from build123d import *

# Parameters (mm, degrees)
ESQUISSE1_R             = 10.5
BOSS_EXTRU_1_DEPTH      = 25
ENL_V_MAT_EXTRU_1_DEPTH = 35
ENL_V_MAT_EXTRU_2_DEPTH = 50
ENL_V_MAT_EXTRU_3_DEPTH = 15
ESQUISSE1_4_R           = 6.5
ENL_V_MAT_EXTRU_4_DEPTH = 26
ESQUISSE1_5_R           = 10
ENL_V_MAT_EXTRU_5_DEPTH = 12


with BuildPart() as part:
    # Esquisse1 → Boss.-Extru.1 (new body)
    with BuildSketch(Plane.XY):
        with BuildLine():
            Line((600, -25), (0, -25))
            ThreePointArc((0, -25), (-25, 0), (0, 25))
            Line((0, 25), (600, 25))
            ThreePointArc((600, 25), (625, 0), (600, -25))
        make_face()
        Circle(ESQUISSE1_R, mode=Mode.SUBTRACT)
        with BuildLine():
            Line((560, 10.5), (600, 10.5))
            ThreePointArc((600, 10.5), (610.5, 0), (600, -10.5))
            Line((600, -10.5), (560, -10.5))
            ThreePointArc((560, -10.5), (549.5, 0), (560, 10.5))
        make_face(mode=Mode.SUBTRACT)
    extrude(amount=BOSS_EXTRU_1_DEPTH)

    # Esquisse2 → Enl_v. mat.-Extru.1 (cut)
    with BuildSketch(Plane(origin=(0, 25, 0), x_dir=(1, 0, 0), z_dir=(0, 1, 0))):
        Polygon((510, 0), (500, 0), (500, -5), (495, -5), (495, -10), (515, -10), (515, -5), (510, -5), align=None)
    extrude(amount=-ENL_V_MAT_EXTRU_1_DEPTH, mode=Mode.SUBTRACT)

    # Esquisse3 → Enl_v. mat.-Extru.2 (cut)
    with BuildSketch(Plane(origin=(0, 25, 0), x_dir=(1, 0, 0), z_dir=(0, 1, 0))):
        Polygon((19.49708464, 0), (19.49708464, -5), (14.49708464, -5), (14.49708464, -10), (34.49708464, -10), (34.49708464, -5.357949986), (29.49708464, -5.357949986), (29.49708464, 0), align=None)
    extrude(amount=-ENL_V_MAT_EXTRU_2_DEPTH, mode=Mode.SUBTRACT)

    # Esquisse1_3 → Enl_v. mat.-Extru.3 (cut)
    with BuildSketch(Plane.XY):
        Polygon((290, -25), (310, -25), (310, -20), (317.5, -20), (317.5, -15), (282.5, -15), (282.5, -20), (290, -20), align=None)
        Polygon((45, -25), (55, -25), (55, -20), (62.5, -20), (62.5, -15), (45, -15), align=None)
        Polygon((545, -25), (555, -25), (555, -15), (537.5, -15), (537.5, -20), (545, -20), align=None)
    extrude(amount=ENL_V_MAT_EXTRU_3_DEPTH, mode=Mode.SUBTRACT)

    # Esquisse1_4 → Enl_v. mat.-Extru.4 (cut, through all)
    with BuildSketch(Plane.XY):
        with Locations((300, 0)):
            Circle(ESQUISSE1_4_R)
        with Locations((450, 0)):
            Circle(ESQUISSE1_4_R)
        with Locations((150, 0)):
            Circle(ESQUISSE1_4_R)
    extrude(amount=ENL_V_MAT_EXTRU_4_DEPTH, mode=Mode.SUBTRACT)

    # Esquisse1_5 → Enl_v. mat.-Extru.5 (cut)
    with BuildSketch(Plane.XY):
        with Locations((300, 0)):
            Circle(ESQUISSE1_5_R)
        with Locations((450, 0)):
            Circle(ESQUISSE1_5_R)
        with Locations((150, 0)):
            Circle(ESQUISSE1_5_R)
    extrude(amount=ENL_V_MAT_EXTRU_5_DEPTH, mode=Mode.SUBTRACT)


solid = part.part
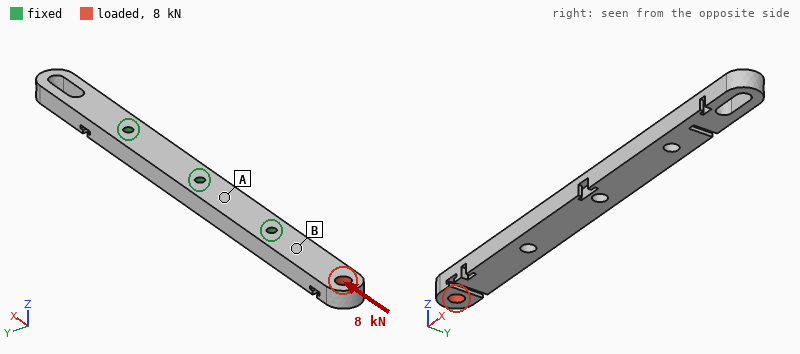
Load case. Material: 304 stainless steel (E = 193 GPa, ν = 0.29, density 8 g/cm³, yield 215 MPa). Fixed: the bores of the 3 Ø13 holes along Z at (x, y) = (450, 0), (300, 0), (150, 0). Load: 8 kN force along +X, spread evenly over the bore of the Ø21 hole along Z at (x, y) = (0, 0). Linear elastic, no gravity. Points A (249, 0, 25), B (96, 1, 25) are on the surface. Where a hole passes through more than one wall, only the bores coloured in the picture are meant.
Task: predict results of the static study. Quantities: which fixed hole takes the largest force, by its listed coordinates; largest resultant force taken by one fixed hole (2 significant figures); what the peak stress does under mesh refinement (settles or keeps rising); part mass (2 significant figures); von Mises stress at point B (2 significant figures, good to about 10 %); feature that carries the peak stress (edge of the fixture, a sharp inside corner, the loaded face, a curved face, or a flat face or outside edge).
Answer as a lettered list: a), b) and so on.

a) (150, 0)
b) 6.8 kN
c) keeps rising
d) 5.8 kg
e) 6.6 MPa
f) edge of the fixture
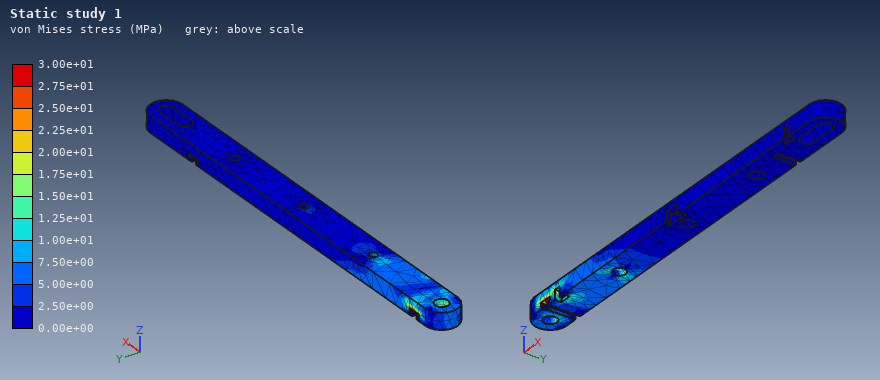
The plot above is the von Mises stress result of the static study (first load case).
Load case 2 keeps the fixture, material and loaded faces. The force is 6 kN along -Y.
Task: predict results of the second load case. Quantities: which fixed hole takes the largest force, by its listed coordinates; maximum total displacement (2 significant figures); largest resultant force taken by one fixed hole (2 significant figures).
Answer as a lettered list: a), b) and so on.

a) (150, 0)
b) 0.30 mm
c) 10 kN
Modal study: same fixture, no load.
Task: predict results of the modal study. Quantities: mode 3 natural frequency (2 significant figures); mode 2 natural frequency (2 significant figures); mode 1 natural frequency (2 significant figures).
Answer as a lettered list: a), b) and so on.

a) 1100 Hz
b) 620 Hz
c) 600 Hz
